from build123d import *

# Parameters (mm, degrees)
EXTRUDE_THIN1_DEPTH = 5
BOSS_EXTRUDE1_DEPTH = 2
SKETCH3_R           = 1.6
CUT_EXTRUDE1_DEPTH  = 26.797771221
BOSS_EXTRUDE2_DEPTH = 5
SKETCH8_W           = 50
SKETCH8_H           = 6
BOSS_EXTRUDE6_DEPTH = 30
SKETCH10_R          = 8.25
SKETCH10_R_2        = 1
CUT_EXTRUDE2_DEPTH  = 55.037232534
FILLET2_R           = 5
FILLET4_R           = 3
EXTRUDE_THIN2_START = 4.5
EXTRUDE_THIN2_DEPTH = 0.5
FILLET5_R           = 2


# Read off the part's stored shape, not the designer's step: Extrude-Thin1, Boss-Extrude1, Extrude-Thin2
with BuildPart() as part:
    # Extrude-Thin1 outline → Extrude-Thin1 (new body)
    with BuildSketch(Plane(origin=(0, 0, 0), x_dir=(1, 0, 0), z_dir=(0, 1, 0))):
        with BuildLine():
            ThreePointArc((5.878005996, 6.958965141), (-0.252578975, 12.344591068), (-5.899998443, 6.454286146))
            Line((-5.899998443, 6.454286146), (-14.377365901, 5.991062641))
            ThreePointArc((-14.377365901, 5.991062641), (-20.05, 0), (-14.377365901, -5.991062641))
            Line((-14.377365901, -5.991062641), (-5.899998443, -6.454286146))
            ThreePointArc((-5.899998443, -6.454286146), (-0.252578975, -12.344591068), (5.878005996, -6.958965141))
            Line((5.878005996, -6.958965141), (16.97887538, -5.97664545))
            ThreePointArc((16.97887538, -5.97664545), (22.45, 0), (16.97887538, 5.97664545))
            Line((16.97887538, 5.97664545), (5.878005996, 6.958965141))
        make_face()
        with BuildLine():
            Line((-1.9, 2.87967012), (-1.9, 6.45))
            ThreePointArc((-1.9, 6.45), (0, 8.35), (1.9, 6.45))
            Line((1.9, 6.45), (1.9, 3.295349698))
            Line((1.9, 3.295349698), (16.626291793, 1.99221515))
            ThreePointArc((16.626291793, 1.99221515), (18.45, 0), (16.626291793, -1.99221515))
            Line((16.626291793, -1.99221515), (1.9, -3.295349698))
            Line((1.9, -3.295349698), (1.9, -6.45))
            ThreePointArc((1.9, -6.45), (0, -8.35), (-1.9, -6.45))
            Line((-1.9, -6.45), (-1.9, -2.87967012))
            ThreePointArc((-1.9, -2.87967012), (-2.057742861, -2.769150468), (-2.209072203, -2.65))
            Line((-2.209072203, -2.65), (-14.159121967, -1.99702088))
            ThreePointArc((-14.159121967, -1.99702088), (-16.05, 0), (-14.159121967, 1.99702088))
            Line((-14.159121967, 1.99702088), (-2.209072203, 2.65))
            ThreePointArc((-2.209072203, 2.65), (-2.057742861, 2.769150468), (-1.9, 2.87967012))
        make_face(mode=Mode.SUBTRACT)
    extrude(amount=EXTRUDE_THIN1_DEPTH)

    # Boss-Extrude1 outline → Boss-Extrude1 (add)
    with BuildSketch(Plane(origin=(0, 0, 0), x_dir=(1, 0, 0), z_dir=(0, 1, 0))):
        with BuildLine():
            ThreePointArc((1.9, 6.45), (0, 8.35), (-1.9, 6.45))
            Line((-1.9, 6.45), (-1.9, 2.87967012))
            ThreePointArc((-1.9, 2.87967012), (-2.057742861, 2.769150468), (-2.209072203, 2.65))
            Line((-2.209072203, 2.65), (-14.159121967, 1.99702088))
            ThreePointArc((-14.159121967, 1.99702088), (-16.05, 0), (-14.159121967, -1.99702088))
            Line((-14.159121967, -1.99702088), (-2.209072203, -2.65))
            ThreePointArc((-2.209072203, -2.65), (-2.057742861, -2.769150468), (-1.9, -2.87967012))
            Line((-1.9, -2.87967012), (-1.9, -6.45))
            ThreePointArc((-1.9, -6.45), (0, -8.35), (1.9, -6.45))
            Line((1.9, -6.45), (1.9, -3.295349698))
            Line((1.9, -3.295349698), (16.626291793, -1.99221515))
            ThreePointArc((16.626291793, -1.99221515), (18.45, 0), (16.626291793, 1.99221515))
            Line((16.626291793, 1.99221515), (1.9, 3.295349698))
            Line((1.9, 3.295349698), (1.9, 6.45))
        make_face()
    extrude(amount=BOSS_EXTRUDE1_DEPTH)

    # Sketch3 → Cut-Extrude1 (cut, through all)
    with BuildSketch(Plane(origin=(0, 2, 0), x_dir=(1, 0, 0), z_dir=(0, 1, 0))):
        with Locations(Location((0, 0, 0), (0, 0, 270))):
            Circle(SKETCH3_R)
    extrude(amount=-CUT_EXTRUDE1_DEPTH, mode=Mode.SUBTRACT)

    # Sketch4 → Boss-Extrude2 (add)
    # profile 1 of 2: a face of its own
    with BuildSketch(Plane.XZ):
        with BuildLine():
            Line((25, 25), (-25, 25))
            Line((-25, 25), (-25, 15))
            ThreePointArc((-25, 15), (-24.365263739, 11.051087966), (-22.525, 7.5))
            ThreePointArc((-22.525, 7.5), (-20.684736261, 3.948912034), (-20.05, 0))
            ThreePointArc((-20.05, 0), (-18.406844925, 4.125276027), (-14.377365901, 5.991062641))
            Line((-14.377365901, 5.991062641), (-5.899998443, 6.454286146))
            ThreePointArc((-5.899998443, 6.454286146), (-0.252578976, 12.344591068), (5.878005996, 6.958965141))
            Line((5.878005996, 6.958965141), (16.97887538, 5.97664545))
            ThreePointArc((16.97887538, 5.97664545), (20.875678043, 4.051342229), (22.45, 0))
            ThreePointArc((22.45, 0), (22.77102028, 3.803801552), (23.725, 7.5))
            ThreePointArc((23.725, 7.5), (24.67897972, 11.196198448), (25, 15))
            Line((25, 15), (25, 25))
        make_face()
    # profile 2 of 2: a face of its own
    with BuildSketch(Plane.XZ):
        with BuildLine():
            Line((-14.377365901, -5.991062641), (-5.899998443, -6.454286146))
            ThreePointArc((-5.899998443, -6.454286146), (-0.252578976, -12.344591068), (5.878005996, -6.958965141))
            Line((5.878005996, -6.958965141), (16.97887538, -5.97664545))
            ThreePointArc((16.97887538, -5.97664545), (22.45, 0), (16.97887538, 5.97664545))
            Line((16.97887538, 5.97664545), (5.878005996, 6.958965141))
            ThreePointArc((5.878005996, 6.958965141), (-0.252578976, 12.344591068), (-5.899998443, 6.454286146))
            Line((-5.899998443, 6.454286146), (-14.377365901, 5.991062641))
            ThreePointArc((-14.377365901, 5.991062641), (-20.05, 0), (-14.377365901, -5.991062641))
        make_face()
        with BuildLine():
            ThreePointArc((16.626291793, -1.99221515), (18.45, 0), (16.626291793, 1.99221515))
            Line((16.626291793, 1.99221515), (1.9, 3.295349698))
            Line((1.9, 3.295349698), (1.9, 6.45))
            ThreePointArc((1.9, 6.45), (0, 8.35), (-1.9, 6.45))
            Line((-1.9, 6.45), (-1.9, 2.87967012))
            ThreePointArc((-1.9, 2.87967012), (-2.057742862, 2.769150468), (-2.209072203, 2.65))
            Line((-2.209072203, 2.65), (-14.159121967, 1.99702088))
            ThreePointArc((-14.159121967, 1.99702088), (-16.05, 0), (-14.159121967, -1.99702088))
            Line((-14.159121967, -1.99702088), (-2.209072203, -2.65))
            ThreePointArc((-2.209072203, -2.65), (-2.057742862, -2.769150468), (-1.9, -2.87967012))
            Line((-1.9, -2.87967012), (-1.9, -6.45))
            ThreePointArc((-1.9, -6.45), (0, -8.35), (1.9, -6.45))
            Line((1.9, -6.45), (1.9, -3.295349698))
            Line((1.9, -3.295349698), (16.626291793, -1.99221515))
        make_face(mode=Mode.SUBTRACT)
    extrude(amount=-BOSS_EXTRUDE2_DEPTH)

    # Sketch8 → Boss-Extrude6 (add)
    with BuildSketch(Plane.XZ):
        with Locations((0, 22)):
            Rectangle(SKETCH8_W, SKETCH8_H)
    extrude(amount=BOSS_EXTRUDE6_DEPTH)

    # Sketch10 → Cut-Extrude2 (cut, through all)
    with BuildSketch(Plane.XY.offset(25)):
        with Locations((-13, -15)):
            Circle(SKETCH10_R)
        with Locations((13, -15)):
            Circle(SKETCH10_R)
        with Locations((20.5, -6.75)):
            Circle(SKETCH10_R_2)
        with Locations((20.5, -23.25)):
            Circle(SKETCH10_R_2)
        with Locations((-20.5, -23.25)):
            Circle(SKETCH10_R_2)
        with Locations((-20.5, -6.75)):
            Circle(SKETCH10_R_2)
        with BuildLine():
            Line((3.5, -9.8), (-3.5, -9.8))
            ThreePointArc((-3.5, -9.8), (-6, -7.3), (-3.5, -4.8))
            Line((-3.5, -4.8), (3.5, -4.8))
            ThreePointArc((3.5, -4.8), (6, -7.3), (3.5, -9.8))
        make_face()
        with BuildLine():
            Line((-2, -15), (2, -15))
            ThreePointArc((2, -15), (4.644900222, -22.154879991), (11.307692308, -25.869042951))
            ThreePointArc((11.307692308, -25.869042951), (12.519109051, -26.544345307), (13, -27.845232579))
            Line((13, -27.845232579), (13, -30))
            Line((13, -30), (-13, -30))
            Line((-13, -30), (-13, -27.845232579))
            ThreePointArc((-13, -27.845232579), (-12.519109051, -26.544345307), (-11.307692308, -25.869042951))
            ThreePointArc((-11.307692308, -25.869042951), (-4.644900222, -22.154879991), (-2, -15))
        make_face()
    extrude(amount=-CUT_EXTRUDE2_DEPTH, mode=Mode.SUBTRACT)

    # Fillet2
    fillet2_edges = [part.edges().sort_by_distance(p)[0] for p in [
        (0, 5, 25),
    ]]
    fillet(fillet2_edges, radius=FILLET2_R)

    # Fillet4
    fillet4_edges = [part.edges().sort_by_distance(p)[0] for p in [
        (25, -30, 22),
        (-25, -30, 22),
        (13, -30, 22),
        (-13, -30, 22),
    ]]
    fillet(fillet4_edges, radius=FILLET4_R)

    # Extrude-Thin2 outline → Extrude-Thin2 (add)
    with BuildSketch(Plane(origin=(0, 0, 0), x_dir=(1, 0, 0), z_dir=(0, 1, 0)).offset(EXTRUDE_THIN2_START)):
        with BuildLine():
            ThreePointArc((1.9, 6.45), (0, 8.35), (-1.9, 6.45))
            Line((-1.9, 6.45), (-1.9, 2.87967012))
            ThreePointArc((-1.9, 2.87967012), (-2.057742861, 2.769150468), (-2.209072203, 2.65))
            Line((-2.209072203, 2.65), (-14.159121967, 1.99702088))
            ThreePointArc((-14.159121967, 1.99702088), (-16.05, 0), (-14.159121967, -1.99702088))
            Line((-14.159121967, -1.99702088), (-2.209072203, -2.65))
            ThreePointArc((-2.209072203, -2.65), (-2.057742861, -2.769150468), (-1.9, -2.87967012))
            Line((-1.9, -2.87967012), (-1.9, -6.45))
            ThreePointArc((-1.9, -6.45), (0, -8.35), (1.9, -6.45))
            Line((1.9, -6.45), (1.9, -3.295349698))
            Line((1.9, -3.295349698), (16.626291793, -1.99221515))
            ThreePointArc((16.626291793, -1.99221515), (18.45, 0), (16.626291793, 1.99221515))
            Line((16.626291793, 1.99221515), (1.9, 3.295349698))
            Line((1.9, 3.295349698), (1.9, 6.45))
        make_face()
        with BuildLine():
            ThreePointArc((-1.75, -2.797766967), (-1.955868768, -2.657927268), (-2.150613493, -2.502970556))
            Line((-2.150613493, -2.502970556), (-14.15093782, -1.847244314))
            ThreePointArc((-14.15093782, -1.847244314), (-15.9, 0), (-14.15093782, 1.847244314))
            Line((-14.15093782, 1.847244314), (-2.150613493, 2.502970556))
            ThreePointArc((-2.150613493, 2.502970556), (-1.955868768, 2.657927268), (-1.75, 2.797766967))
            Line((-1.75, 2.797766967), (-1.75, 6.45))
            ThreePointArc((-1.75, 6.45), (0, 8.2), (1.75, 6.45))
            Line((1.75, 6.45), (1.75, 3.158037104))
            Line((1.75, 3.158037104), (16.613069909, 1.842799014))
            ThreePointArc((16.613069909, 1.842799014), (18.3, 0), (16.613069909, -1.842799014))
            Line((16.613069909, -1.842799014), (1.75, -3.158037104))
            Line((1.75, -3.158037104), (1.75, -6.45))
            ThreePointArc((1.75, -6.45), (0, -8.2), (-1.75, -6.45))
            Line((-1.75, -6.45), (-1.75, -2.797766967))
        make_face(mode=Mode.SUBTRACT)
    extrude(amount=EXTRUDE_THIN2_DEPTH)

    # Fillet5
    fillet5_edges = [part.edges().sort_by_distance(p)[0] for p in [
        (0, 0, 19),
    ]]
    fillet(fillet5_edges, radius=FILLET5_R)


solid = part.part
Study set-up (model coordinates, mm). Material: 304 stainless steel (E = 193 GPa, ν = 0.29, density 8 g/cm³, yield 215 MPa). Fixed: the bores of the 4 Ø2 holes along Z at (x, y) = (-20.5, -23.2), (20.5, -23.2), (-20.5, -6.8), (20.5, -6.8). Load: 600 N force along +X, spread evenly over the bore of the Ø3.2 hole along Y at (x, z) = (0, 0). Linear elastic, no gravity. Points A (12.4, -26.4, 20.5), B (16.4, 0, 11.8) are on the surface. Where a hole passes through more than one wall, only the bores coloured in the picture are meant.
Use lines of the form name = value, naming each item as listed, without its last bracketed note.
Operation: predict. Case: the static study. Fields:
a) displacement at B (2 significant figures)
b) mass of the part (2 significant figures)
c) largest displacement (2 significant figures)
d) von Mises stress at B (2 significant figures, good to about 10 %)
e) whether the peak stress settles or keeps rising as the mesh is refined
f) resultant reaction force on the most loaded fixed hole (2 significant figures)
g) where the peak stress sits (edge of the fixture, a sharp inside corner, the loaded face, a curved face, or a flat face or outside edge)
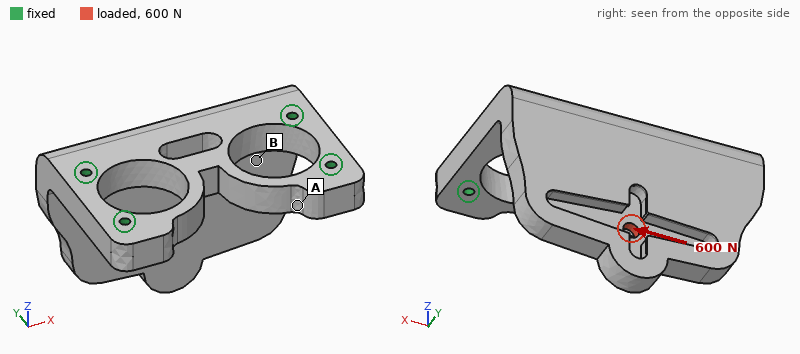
displacement at B = 3.3 µm
mass of the part = 92 g
largest displacement = 7.1 µm
von Mises stress at B = 11 MPa
whether the peak stress settles or keeps rising as the mesh is refined = keeps rising
resultant reaction force on the most loaded fixed hole = 450 N
where the peak stress sits = edge of the fixture
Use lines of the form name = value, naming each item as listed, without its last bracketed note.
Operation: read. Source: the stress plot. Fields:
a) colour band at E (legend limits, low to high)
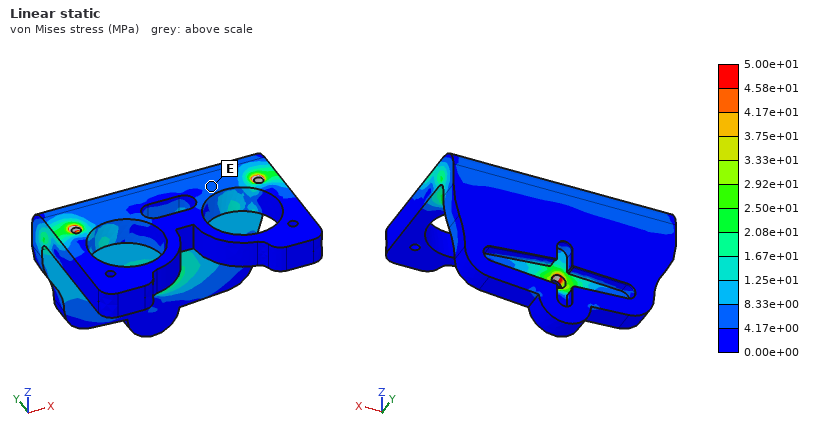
colour band at E = 4.17e+00 to 8.33e+00 MPa
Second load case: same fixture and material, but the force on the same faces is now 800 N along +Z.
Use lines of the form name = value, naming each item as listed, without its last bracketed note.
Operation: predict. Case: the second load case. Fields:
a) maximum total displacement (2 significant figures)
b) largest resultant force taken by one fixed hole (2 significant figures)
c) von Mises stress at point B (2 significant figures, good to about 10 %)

maximum total displacement = 10 µm
largest resultant force taken by one fixed hole = 430 N
von Mises stress at point B = 11 MPa
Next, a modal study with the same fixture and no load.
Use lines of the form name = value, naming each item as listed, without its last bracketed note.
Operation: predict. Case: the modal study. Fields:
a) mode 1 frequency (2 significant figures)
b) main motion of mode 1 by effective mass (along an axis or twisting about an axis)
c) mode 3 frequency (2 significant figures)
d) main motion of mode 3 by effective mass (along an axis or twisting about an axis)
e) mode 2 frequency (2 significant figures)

mode 1 frequency = 3300 Hz
main motion of mode 1 by effective mass = along Y
mode 3 frequency = 10 kHz
main motion of mode 3 by effective mass = along Z
mode 2 frequency = 7800 Hz
